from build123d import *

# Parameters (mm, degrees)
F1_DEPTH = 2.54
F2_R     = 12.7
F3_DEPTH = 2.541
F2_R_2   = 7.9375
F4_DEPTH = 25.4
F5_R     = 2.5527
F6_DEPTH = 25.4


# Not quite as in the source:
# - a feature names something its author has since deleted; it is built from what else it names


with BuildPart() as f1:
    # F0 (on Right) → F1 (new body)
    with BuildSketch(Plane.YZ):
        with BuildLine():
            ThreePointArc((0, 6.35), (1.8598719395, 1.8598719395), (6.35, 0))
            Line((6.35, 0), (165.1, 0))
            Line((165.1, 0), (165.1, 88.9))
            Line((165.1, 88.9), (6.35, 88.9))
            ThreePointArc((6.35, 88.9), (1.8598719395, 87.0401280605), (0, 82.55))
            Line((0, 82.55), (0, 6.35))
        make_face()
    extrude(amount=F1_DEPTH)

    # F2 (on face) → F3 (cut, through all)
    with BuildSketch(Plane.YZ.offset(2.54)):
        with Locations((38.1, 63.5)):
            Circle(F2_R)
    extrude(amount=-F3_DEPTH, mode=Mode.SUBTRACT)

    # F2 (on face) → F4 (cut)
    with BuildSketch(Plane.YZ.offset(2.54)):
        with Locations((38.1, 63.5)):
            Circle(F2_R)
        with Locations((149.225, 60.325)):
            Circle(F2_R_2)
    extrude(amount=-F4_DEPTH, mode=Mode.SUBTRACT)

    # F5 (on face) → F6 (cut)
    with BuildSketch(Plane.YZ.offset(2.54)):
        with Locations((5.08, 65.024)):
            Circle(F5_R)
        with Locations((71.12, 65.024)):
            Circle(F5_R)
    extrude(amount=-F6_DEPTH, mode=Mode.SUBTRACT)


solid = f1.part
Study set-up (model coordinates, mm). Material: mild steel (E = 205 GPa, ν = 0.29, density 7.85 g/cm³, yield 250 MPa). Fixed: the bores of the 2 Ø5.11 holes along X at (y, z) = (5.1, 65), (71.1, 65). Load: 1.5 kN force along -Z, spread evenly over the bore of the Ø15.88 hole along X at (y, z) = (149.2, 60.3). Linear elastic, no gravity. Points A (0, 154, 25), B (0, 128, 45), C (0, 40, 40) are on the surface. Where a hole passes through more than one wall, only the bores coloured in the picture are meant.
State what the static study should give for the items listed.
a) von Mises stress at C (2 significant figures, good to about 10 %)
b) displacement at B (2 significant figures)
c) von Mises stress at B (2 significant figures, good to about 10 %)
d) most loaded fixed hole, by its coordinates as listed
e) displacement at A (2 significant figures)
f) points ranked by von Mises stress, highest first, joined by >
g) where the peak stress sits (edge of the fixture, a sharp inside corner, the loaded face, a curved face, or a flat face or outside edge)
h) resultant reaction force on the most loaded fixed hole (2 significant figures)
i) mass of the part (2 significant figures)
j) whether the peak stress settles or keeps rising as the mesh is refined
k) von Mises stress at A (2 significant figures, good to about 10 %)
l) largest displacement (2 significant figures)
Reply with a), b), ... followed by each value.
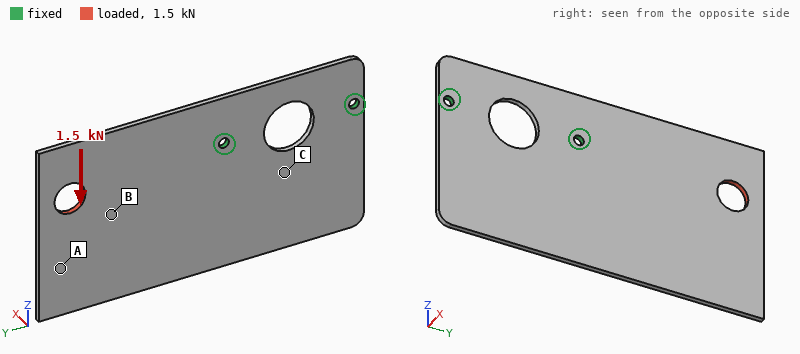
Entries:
a) 30 MPa
b) 32 µm
c) 17 MPa
d) (71.1, 65)
e) 47 µm
f) C > B > A
g) edge of the fixture
h) 3.2 kN
i) 280 g
j) keeps rising
k) 7.8 MPa
l) 56 µm
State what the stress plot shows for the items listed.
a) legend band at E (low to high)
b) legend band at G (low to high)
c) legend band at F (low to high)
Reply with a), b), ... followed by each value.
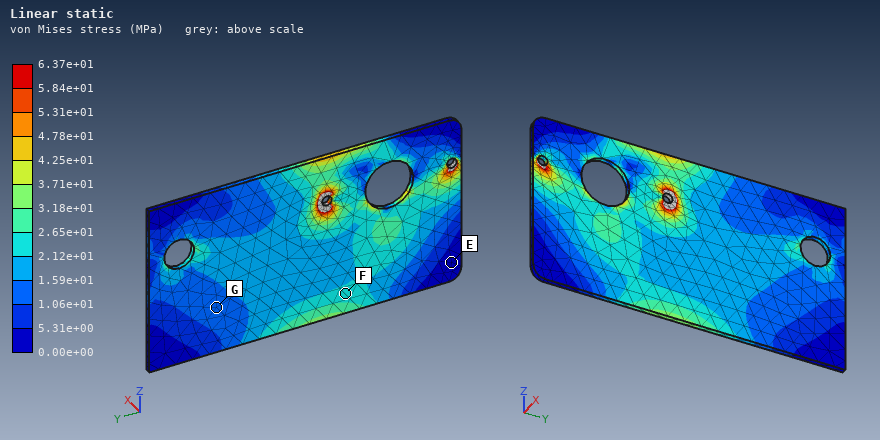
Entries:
a) 0.00e+00 to 5.31e+00 MPa
b) 1.06e+01 to 1.59e+01 MPa
c) 2.12e+01 to 2.65e+01 MPa
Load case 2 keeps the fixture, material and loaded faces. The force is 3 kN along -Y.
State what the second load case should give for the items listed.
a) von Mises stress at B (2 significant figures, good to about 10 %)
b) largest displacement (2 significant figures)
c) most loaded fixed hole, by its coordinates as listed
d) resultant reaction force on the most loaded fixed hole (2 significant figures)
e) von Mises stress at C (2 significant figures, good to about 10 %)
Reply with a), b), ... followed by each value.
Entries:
a) 20 MPa
b) 15 µm
c) (71.1, 65)
d) 2.5 kN
e) 7.7 MPa
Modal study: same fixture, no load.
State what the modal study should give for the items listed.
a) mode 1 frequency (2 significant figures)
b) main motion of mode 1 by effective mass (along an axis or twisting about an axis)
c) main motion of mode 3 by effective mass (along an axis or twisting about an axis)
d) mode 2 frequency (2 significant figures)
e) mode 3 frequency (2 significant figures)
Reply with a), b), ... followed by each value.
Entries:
a) 200 Hz
b) along X
c) along X
d) 370 Hz
e) 610 Hz
